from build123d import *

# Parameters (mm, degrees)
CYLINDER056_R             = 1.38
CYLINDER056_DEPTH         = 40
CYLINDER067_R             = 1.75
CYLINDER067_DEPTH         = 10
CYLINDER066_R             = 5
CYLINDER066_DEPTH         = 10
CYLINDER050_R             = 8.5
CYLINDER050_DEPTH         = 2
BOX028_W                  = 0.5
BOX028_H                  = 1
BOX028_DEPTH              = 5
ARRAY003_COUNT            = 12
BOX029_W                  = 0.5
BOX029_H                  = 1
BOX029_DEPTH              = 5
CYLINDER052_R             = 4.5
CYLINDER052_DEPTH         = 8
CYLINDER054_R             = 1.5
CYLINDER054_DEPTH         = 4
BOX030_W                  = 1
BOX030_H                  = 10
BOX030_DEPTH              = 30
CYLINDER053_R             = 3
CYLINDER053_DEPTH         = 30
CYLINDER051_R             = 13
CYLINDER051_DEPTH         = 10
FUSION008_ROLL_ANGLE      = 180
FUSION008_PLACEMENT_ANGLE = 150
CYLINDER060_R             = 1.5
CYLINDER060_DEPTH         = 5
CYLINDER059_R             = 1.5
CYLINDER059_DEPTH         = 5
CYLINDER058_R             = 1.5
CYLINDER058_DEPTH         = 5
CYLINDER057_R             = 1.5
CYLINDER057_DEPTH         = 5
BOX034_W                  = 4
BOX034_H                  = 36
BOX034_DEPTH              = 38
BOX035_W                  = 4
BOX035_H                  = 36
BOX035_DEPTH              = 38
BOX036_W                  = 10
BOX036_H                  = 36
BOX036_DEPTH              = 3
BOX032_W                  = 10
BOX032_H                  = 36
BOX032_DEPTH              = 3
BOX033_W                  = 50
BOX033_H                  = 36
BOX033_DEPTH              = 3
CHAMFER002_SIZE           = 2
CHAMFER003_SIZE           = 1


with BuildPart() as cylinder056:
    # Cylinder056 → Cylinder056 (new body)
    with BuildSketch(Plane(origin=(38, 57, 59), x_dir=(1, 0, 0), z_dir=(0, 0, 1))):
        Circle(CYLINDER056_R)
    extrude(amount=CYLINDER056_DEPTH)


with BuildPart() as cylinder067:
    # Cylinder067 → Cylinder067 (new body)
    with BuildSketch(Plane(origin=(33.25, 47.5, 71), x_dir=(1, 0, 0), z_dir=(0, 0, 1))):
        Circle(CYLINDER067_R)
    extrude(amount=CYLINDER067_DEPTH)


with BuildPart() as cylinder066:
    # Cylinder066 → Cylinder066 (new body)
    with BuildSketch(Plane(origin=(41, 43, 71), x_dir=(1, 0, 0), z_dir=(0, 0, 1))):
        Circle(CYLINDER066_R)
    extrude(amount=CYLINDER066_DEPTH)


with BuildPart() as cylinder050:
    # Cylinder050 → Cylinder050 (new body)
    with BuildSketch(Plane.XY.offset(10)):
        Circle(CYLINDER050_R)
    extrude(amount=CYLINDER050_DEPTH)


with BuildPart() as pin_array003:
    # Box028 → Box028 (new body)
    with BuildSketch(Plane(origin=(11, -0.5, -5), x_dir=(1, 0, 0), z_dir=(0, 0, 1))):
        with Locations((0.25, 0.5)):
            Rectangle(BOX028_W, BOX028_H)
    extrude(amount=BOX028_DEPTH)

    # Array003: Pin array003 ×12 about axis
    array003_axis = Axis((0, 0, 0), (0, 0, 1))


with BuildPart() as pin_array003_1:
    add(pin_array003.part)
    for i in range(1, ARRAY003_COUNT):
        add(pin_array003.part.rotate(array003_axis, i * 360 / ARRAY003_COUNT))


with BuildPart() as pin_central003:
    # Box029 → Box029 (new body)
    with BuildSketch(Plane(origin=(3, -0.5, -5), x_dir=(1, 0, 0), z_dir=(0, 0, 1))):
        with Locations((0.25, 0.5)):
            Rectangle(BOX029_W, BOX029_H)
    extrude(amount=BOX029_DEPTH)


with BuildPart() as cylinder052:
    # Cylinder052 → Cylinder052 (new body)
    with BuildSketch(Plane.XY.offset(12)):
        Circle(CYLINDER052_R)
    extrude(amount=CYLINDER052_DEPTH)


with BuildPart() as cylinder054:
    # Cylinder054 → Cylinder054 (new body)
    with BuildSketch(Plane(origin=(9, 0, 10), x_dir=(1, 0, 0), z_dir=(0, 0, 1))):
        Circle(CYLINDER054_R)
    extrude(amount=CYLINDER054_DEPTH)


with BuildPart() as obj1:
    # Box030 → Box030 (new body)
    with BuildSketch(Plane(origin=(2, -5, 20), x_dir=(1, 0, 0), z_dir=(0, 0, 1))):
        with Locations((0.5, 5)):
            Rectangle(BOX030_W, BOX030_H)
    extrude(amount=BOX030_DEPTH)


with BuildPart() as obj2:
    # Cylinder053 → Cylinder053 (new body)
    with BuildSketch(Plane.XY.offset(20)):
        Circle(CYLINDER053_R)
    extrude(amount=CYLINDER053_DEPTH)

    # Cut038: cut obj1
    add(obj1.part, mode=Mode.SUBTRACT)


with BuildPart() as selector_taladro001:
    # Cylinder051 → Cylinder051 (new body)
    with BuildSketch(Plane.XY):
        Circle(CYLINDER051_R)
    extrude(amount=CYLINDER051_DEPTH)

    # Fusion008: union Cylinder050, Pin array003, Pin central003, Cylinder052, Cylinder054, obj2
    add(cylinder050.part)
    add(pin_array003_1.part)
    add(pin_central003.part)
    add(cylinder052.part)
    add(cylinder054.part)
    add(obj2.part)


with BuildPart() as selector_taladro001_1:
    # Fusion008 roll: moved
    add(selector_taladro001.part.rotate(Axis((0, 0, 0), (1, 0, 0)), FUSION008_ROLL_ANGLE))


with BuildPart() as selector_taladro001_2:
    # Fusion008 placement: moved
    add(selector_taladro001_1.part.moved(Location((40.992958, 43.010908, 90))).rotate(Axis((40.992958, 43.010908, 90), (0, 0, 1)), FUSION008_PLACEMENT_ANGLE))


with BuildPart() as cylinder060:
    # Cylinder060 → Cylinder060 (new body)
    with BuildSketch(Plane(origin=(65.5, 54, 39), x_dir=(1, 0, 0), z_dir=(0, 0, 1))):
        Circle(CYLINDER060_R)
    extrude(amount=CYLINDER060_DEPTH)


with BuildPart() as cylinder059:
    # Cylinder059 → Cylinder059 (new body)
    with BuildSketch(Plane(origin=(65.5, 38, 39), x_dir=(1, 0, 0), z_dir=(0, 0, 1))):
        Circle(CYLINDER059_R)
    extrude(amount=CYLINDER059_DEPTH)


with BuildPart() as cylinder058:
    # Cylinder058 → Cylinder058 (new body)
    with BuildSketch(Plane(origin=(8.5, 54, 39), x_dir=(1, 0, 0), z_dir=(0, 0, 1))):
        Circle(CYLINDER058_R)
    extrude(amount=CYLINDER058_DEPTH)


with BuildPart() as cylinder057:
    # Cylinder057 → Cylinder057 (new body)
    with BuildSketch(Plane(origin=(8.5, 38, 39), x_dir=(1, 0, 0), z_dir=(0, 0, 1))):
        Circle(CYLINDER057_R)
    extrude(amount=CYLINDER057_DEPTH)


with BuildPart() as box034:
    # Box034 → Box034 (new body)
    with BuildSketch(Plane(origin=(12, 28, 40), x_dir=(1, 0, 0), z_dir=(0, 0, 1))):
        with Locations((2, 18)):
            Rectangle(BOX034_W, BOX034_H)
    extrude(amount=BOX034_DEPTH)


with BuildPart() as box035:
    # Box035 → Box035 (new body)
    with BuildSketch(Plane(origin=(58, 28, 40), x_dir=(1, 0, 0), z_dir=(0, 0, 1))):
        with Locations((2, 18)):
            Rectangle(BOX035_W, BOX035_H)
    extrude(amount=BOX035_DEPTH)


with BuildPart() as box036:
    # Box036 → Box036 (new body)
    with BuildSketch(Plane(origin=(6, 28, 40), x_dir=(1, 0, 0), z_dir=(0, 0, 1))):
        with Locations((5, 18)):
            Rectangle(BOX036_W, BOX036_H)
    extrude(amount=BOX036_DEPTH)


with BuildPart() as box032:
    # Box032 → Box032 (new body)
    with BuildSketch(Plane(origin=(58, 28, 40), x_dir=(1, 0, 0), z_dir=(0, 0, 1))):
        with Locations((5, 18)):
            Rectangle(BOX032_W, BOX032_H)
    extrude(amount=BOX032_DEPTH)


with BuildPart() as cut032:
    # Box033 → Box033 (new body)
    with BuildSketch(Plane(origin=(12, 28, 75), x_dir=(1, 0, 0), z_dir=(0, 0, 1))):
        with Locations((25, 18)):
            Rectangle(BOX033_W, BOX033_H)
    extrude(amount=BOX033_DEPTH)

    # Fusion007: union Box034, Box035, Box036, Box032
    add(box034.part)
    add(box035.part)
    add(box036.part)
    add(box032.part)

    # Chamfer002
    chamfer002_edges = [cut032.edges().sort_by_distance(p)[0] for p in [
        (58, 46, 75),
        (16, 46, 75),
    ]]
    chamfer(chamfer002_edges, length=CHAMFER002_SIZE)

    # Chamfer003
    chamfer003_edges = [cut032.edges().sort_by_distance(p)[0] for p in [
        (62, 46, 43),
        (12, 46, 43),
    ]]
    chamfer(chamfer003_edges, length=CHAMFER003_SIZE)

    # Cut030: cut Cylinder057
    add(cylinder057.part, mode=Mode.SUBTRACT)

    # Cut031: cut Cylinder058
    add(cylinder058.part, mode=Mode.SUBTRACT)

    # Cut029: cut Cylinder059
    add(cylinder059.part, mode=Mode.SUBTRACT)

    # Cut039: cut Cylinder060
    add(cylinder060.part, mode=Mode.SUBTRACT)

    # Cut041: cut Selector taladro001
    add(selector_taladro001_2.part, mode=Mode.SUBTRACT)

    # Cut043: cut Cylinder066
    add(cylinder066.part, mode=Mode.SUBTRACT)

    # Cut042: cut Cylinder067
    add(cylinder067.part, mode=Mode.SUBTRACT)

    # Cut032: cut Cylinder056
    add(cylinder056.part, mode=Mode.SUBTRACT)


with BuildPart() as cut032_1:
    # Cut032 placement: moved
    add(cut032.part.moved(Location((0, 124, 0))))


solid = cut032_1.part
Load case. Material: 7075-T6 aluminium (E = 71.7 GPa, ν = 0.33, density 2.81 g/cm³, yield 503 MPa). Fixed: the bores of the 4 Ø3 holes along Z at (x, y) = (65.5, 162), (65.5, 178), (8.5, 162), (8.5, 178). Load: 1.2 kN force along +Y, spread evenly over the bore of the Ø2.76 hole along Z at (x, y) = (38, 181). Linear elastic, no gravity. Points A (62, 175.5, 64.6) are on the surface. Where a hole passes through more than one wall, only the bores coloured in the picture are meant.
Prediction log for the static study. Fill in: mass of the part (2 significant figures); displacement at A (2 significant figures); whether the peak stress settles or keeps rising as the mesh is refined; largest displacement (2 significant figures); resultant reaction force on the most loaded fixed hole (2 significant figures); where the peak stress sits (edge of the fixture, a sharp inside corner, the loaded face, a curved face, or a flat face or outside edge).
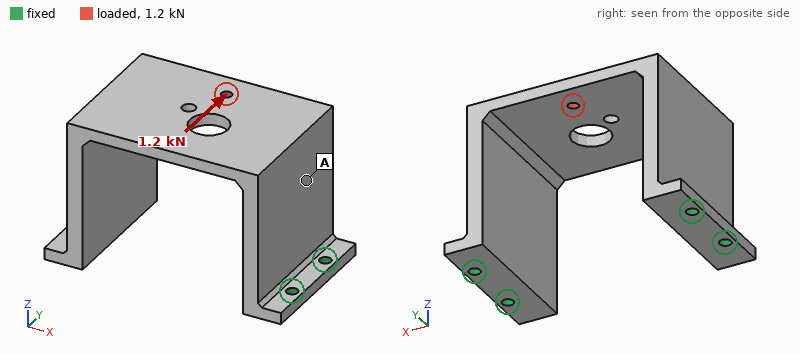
47 g
56 µm
keeps rising
98 µm
1.2 kN
edge of the fixture
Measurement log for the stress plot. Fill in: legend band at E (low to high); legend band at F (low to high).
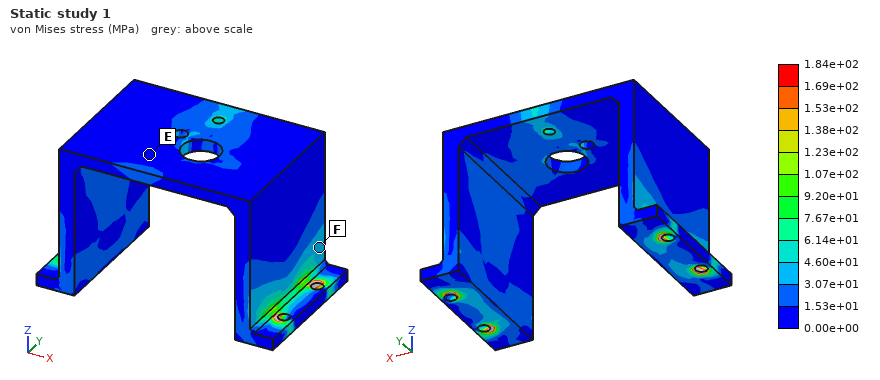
0.00e+00 to 1.53e+01 MPa
3.07e+01 to 4.60e+01 MPa
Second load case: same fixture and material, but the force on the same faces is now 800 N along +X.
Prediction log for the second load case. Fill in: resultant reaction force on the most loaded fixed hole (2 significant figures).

520 N
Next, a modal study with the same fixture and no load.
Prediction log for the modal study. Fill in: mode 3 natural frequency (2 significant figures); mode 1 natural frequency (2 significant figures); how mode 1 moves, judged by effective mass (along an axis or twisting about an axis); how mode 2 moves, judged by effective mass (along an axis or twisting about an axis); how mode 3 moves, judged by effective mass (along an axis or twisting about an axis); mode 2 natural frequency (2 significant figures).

4100 Hz
1800 Hz
along X
along Y
twisting about Z
3800 Hz
